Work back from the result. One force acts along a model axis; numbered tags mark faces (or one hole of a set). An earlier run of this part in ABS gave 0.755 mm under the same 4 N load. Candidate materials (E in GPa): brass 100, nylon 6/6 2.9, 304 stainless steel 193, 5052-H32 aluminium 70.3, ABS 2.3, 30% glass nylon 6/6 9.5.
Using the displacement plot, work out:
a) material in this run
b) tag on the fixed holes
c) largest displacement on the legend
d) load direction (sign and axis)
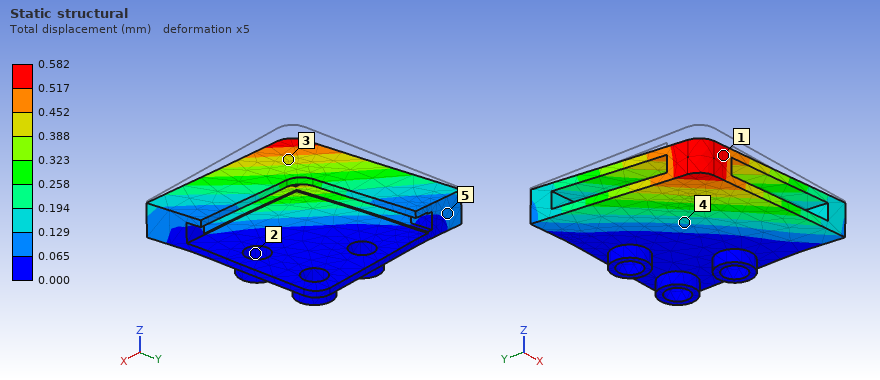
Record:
nylon 6/6
2
0.582 mm
-Z
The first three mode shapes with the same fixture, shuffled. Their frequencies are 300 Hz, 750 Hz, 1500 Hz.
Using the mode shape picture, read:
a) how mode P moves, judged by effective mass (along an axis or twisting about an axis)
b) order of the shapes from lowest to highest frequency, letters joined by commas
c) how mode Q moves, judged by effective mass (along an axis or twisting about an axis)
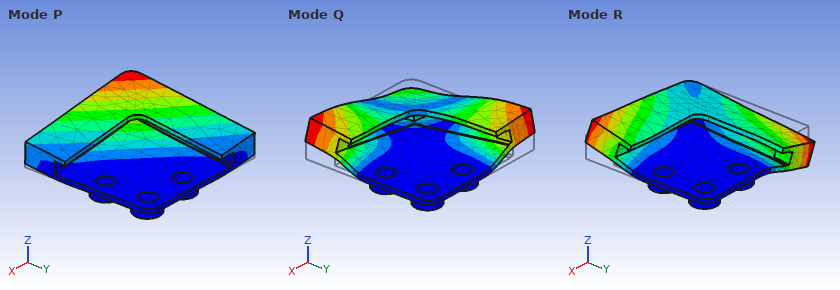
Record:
along Z
P, R, Q
along Z
